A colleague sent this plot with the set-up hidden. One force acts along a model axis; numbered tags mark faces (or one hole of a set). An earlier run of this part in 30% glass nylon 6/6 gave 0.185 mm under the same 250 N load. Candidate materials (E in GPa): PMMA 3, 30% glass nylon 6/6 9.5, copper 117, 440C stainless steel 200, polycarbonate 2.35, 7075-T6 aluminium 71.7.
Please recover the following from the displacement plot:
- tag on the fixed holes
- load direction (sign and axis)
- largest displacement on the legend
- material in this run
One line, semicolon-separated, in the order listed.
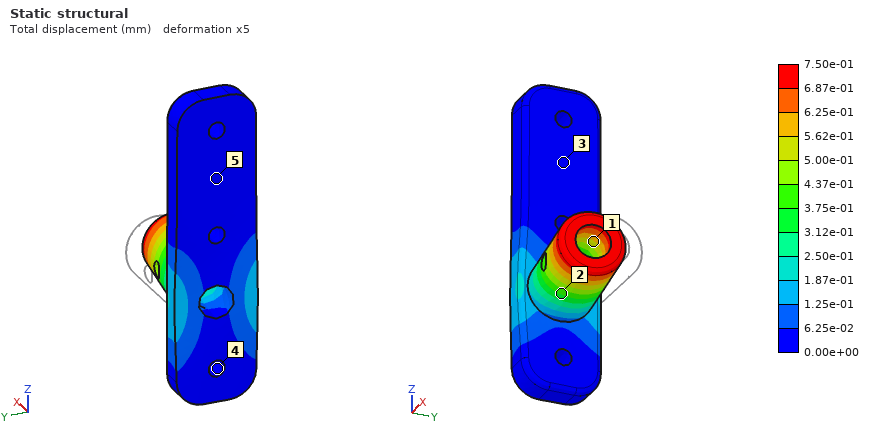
4; -Y; 7.50e-01 mm; polycarbonate
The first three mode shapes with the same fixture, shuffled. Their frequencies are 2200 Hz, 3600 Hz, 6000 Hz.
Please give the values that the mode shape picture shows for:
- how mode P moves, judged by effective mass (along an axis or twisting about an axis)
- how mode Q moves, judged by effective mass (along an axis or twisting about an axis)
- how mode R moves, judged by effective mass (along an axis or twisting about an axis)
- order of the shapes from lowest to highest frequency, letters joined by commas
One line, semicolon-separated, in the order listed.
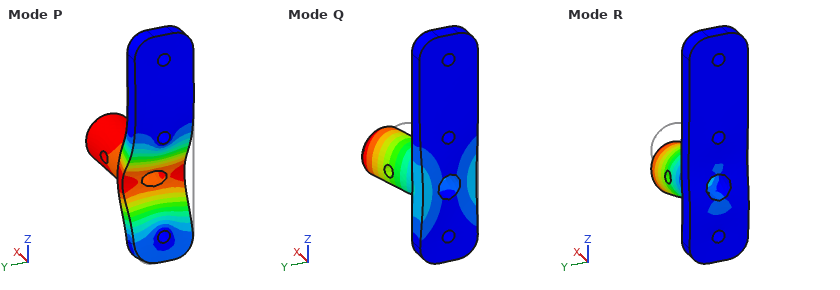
along X; along Y; along Z; Q, R, P
